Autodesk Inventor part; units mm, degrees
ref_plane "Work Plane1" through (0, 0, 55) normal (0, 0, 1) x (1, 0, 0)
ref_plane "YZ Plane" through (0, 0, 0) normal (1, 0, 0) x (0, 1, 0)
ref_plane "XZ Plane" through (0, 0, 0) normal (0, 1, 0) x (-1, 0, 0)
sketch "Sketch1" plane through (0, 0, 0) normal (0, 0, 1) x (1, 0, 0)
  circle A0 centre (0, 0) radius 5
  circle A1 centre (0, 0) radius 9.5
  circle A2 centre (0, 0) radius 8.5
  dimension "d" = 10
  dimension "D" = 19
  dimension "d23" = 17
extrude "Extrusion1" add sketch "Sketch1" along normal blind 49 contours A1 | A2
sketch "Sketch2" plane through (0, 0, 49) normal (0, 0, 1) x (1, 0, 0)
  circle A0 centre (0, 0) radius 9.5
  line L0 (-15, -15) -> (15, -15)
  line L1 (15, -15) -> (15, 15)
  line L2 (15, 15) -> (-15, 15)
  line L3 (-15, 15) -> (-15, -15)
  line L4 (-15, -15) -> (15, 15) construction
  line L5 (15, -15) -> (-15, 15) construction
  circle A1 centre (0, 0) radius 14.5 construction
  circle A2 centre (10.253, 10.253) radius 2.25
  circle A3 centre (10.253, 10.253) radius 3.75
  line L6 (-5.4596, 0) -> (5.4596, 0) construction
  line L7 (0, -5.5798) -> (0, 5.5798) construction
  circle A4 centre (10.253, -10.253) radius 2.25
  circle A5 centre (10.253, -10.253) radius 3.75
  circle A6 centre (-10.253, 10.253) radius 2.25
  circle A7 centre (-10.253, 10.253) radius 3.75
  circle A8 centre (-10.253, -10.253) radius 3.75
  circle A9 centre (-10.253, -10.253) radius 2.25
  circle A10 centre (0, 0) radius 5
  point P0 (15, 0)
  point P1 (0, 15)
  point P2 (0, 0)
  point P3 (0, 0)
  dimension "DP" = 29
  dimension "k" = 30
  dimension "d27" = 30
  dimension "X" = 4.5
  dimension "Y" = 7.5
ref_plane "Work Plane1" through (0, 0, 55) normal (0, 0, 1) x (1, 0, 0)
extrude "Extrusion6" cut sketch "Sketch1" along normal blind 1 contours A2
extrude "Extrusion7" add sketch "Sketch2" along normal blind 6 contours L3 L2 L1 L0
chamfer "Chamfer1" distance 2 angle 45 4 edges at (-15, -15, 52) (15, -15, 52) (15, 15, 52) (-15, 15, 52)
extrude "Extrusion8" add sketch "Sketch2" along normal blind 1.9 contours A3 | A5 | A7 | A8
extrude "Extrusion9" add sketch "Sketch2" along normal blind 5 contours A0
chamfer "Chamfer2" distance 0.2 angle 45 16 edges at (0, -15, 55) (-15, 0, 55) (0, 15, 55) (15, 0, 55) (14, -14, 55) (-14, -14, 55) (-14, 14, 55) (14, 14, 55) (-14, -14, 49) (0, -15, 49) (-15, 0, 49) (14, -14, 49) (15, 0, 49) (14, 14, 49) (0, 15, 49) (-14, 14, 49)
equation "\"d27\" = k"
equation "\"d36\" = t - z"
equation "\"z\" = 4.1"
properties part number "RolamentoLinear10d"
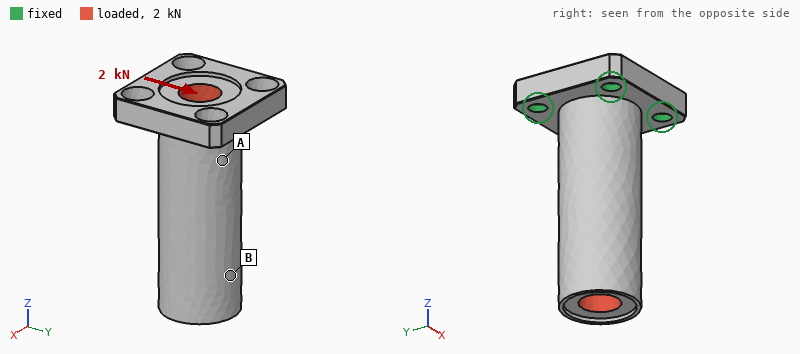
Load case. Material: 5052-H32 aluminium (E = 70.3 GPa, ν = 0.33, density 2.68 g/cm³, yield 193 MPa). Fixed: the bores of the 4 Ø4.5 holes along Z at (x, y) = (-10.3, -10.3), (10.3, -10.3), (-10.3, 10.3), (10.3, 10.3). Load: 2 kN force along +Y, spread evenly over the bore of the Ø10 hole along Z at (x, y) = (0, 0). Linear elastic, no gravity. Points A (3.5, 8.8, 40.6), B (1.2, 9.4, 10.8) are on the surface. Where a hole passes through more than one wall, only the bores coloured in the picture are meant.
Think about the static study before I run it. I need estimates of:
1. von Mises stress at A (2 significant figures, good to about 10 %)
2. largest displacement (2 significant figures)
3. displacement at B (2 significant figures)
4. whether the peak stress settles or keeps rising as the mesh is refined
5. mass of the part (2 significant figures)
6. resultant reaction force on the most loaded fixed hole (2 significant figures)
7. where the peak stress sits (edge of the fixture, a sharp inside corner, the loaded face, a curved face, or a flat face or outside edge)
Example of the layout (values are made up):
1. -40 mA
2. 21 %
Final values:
1. 42 MPa
2. 0.16 mm
3. 0.13 mm
4. keeps rising
5. 37 g
6. 1.3 kN
7. edge of the fixture
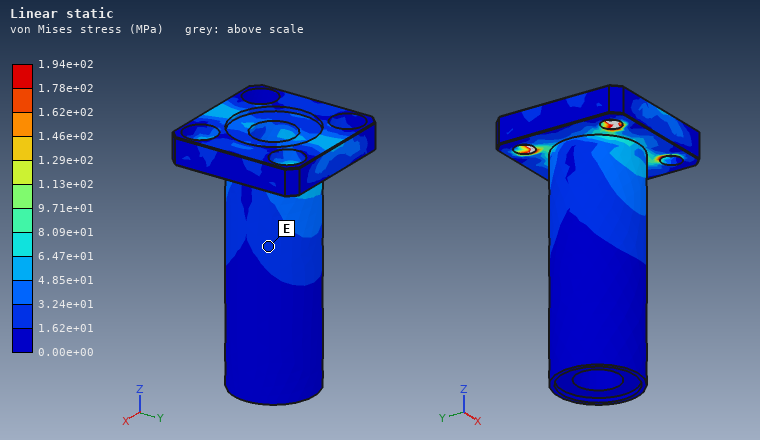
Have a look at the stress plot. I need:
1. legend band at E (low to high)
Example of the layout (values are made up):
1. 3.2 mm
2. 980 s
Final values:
1. 1.62e+01 to 3.24e+01 MPa
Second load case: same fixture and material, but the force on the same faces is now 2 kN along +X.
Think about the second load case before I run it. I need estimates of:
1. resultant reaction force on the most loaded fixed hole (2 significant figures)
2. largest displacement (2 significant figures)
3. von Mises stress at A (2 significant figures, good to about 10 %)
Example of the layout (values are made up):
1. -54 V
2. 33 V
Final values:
1. 1.3 kN
2. 0.16 mm
3. 22 MPa
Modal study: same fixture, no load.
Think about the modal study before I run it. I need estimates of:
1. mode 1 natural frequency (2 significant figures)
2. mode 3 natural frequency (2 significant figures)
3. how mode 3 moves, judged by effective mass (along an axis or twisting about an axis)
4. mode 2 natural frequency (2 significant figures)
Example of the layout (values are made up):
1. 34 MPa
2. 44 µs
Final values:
1. 4000 Hz
2. 15 kHz
3. along Z
4. 4000 Hz
